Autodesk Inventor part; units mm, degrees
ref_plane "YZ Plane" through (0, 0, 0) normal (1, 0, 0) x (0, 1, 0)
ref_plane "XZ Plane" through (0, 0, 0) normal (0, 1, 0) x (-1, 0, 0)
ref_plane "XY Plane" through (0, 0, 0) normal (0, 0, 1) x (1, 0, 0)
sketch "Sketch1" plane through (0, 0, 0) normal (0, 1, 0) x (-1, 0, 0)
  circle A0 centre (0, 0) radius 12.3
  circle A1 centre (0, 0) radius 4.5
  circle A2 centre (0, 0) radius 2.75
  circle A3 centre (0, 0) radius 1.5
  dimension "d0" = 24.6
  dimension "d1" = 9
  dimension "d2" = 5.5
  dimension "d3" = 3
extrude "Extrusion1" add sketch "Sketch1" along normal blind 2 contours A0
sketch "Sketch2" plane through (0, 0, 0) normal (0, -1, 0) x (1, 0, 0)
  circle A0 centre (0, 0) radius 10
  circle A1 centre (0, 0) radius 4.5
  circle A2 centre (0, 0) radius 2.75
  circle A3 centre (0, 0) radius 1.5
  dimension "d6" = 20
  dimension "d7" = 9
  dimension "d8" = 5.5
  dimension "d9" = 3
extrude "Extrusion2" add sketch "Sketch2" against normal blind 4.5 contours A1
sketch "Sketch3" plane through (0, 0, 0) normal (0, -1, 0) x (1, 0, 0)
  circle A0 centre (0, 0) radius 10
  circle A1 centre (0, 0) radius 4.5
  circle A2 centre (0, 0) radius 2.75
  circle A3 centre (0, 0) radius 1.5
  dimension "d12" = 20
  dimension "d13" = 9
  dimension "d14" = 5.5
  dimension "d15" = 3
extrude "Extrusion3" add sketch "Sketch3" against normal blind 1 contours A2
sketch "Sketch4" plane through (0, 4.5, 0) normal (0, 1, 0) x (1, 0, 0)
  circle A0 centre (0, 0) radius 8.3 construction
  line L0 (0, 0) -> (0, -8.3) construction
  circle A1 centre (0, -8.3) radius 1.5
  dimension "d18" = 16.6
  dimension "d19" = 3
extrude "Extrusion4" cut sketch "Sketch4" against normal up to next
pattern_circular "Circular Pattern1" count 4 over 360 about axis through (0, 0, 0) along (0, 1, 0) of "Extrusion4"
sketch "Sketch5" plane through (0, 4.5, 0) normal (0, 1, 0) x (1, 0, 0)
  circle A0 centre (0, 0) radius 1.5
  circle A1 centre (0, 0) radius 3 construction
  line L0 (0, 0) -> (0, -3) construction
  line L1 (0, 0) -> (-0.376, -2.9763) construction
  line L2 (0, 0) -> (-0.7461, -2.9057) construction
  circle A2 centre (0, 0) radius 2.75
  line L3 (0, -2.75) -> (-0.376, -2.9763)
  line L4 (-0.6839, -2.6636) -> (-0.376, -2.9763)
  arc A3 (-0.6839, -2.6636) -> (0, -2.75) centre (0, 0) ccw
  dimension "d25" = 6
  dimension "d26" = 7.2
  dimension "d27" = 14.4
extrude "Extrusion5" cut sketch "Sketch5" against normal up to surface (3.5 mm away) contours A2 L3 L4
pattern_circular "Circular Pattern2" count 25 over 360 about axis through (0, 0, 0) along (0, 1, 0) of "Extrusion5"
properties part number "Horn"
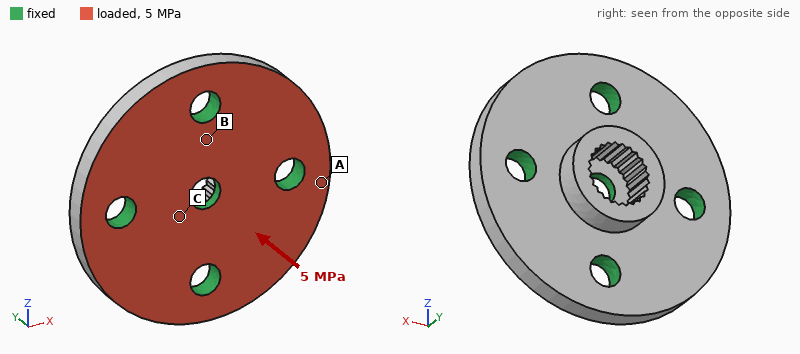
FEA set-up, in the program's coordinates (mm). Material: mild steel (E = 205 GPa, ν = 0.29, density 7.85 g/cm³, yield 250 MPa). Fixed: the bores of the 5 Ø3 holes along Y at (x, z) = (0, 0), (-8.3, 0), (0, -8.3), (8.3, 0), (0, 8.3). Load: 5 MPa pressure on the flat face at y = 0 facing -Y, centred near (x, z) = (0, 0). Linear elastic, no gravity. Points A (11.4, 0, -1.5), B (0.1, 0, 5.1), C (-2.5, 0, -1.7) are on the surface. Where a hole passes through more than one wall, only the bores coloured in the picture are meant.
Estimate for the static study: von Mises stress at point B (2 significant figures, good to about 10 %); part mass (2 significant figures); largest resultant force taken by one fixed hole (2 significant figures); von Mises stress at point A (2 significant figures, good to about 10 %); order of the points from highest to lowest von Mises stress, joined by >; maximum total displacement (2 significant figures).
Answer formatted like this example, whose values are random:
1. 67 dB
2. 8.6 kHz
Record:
1. 29 MPa
2. 7.5 g
3. 500 N
4. 49 MPa
5. A > B > C
6. 5.9 µm
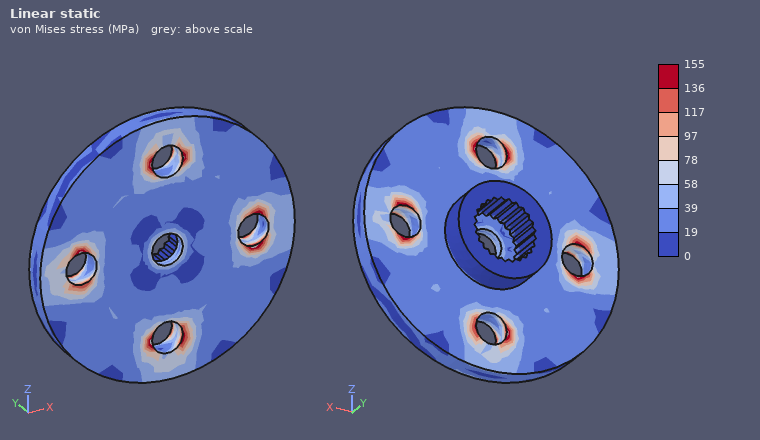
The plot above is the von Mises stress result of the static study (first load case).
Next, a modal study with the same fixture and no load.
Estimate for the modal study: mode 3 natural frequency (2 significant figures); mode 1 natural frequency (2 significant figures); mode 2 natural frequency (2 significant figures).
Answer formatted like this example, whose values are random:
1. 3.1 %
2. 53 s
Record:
1. 49 kHz
2. 47 kHz
3. 49 kHz
